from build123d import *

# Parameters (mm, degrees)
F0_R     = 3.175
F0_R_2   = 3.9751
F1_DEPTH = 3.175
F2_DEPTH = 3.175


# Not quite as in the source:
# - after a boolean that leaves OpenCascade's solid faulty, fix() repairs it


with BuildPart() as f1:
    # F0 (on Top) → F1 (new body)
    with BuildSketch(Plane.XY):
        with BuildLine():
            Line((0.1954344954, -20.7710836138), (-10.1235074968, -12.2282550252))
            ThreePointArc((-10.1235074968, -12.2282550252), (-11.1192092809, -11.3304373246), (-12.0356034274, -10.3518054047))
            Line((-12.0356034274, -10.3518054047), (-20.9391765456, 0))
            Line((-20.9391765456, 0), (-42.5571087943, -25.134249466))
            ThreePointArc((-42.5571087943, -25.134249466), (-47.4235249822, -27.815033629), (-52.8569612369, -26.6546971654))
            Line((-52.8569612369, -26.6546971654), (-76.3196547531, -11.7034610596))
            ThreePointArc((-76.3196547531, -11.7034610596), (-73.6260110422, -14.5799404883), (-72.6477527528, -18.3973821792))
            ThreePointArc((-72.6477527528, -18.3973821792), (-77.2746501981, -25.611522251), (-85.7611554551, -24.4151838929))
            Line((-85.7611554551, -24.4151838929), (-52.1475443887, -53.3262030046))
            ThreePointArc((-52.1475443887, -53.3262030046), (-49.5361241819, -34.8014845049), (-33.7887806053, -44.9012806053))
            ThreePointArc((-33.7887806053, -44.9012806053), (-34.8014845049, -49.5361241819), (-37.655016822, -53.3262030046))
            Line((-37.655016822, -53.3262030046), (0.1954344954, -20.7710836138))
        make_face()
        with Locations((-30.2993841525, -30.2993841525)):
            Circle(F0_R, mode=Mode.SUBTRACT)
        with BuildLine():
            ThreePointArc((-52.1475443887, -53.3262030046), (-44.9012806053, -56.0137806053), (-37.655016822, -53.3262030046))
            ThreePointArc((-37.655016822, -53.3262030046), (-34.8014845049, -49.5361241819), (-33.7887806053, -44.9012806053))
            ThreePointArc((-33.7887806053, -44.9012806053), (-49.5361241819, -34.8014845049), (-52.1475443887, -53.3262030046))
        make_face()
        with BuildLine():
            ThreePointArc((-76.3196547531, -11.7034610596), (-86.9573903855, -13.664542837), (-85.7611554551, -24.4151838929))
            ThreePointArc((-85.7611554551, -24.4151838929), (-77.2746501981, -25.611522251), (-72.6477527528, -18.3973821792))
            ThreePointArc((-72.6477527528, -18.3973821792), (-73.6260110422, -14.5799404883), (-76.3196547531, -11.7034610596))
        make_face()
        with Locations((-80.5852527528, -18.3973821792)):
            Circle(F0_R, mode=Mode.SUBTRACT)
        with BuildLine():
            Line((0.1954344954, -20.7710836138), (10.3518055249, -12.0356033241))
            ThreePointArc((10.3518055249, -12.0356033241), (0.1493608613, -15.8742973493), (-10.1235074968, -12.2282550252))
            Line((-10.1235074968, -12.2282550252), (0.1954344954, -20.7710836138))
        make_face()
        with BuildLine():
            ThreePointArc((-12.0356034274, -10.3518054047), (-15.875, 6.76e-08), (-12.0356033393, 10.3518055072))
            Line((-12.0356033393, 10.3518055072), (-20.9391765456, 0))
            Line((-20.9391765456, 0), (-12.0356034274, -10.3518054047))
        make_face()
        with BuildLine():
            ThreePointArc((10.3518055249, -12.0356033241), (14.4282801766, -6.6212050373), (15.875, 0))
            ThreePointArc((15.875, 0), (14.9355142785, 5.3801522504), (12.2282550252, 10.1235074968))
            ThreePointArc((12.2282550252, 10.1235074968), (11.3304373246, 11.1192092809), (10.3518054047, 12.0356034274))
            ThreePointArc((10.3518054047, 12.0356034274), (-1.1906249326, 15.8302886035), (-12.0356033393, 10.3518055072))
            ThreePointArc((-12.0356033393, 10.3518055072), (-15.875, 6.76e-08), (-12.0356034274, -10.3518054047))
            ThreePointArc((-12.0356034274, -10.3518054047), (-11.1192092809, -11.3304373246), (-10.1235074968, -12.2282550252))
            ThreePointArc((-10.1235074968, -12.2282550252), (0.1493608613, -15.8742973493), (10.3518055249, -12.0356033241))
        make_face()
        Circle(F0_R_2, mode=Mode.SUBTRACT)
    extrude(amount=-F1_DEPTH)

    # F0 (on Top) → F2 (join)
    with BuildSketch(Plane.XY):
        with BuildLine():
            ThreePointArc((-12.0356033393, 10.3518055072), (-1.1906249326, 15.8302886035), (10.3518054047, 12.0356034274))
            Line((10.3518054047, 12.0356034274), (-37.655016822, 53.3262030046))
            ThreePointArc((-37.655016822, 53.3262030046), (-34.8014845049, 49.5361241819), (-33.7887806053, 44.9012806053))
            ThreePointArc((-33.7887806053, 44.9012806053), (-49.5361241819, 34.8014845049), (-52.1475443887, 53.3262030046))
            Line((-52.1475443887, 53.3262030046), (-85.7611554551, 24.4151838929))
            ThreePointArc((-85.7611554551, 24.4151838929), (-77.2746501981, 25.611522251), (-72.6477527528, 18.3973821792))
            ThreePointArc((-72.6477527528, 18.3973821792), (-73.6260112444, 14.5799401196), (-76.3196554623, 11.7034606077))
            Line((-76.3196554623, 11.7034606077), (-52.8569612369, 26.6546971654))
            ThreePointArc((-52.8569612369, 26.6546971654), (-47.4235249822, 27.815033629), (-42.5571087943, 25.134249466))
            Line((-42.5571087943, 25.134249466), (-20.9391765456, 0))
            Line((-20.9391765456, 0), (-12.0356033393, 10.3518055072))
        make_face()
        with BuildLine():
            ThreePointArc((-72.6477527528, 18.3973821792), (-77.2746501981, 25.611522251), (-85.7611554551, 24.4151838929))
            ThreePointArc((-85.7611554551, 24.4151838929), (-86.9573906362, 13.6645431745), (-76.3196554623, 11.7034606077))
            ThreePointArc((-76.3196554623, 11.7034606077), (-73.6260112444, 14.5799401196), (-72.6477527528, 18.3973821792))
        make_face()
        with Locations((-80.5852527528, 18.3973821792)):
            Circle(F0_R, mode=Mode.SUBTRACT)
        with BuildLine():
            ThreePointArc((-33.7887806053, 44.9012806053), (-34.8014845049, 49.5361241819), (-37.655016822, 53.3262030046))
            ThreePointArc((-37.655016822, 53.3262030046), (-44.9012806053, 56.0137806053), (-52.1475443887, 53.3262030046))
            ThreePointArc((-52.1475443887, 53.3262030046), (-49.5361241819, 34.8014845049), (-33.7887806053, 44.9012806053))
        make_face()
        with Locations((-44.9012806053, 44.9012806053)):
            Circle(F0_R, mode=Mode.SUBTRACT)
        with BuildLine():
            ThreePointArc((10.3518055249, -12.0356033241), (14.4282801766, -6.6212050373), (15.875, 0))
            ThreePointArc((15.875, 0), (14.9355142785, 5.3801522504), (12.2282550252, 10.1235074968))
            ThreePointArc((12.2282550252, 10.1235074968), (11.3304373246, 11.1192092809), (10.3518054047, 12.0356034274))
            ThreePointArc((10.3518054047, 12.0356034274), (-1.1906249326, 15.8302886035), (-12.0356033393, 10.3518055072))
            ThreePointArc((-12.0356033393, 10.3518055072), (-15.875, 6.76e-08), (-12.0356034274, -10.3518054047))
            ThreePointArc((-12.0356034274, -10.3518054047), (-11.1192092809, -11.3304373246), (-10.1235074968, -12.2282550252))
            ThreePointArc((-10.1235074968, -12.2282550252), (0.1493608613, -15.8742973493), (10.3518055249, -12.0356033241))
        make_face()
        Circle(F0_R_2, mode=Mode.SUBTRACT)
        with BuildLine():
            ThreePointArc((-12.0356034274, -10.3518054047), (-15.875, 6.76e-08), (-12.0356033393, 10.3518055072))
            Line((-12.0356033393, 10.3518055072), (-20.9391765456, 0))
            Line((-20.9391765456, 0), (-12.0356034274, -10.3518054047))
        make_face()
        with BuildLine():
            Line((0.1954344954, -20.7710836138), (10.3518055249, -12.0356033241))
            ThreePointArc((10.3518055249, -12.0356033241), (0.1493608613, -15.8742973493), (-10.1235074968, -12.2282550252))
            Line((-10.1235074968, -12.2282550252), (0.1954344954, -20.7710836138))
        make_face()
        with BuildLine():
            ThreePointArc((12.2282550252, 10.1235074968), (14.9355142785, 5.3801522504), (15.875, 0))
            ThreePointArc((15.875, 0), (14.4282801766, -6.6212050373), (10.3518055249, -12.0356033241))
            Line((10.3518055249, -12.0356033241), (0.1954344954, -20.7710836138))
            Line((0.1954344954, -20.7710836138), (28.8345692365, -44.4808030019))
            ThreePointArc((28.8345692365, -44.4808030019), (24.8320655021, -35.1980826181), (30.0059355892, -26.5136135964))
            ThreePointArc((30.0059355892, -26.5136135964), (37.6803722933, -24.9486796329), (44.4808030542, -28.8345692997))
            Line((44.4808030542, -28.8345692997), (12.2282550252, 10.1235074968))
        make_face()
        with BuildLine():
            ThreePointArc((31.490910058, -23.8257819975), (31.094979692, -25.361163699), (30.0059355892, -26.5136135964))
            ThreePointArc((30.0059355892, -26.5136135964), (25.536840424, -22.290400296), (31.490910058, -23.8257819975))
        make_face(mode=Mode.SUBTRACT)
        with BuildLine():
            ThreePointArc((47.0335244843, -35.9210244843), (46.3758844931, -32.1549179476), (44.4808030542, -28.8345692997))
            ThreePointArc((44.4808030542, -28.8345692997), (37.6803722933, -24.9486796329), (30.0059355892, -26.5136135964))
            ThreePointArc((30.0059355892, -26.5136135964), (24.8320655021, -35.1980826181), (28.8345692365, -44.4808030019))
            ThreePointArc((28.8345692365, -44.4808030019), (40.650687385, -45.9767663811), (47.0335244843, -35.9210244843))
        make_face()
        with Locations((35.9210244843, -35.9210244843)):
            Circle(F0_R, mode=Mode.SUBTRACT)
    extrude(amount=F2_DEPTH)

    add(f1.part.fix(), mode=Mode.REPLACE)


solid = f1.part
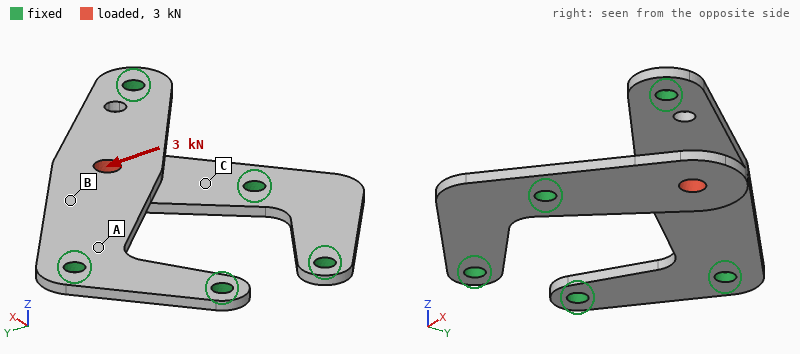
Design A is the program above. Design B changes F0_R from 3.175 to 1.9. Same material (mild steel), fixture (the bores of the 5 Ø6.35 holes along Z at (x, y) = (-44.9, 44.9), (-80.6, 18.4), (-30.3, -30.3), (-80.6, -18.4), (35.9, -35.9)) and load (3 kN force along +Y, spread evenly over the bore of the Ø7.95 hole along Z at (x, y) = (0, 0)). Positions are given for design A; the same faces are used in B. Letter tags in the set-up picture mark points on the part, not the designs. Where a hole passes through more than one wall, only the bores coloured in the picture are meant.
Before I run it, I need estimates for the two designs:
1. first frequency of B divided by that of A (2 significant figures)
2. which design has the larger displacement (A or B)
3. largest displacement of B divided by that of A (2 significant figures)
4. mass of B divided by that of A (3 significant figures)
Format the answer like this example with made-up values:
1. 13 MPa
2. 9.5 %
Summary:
1. 0.93
2. B
3. 1.1
4. 1.01
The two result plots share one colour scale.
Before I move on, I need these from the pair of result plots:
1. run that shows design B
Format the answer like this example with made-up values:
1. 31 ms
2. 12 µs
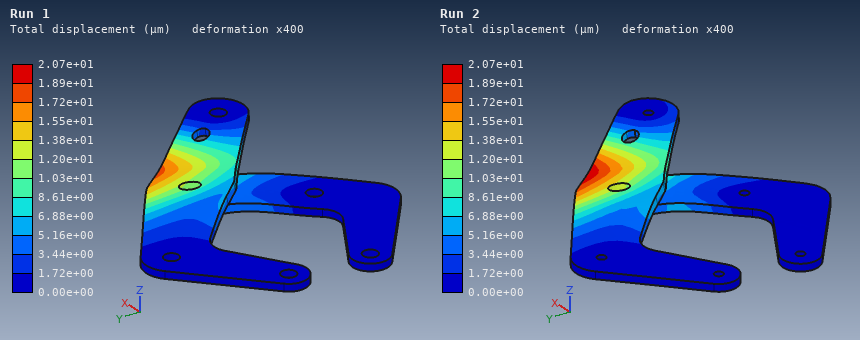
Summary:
1. Run 2
